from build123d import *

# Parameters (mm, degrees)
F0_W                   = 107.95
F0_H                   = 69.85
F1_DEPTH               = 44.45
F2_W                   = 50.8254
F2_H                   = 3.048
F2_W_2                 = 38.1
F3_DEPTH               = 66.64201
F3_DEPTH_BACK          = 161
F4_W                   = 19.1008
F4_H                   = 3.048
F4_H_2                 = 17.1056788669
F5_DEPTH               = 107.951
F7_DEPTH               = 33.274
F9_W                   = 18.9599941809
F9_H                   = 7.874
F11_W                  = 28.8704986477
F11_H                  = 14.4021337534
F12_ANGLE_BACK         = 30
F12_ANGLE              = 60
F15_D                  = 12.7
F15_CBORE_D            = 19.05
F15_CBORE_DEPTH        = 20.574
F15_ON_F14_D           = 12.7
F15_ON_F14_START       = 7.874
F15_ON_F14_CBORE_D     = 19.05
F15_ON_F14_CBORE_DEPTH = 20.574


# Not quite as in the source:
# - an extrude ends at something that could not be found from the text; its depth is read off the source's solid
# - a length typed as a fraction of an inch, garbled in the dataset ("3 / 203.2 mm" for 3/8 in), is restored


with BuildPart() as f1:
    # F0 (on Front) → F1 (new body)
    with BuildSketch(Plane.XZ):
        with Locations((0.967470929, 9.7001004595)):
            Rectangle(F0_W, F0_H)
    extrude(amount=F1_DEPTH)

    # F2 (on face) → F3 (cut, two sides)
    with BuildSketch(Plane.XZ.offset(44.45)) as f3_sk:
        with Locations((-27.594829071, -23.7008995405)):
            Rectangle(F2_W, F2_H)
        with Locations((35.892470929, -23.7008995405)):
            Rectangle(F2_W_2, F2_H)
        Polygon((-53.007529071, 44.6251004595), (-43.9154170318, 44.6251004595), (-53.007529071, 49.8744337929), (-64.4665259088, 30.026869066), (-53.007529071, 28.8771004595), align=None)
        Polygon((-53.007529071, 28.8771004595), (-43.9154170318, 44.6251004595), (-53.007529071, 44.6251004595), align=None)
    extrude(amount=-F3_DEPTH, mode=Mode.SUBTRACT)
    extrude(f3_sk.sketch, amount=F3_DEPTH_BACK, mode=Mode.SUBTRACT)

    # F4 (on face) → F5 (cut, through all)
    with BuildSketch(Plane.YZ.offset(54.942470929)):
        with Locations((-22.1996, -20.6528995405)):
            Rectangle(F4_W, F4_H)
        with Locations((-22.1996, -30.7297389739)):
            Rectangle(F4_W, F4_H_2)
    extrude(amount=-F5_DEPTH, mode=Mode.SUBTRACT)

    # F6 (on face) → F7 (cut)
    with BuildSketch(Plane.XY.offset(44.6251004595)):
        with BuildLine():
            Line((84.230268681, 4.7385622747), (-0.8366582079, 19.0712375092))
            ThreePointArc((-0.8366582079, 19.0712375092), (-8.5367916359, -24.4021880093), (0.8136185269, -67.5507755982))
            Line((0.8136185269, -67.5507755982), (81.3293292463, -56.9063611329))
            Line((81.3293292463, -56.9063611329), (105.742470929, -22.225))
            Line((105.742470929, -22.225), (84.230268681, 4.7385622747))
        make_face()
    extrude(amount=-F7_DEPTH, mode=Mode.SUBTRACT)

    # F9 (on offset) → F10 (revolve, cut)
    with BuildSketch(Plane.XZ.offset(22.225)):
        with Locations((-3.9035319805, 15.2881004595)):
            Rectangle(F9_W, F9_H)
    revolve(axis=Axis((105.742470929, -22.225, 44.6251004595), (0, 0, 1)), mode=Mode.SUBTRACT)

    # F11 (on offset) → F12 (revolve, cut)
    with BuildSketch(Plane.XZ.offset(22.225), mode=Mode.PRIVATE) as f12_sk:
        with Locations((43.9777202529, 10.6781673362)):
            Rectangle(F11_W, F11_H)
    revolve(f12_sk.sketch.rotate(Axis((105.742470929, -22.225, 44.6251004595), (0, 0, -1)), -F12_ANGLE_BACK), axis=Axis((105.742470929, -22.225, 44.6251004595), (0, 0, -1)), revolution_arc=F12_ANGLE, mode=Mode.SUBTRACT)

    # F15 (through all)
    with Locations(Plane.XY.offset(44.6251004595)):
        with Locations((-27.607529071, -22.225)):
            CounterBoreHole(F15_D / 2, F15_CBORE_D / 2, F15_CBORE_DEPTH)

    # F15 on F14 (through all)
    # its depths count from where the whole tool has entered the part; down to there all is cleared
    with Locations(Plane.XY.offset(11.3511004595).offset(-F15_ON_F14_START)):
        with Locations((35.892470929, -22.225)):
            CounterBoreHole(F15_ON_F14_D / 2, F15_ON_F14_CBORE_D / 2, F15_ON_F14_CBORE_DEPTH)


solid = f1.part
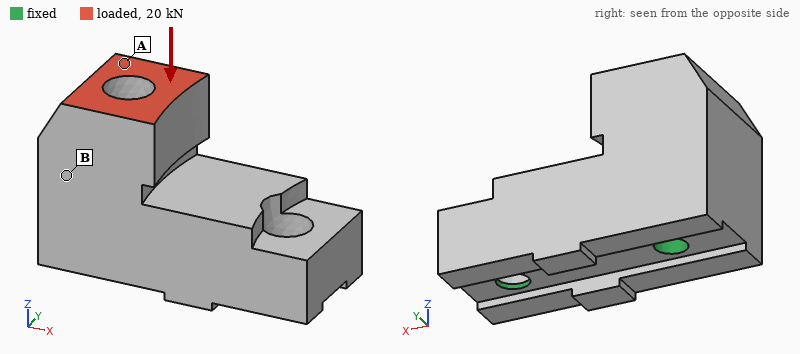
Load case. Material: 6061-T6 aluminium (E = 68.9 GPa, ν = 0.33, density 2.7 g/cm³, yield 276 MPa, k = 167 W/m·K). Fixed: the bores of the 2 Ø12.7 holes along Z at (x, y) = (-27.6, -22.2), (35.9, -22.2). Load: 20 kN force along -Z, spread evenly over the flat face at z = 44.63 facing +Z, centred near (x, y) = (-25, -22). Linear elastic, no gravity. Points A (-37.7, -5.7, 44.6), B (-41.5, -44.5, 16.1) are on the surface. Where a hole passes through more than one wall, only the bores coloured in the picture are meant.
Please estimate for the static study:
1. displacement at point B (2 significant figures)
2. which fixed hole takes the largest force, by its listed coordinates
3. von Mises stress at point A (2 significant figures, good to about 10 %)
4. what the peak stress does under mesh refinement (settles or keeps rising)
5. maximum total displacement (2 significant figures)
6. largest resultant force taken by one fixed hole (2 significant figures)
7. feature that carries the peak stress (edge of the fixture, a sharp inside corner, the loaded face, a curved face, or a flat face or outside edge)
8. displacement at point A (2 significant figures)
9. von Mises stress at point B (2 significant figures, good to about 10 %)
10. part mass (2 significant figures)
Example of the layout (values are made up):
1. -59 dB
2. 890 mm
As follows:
1. 3.6 µm
2. (-27.6, -22.2)
3. 14 MPa
4. keeps rising
5. 16 µm
6. 20 kN
7. edge of the fixture
8. 9.3 µm
9. 5.8 MPa
10. 520 g
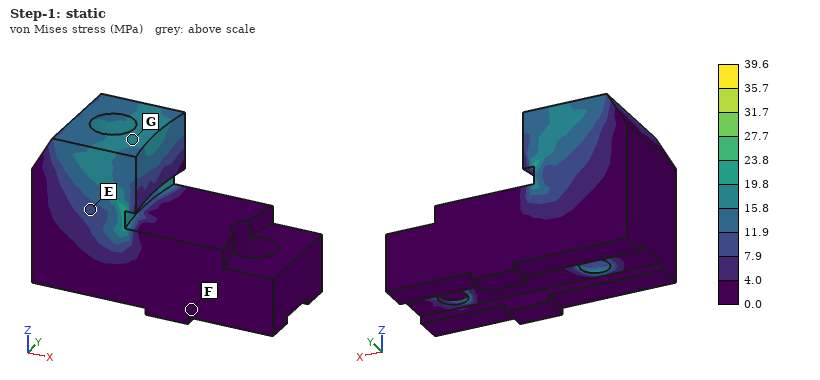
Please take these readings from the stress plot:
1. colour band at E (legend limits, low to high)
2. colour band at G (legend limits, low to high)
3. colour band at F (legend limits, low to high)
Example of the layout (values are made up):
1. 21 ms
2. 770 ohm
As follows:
1. 7.9 to 11.9 MPa
2. 15.8 to 19.8 MPa
3. 0.0 to 4.0 MPa
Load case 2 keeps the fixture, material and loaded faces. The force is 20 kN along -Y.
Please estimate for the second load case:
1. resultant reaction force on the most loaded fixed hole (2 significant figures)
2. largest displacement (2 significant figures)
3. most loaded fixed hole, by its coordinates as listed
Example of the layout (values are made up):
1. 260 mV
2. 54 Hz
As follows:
1. 20 kN
2. 68 µm
3. (-27.6, -22.2)
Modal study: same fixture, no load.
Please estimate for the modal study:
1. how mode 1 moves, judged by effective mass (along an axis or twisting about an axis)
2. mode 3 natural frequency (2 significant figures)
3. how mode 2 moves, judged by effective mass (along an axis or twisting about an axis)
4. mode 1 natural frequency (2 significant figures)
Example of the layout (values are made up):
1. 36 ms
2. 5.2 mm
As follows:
1. along Y
2. 13 kHz
3. along Z
4. 7700 Hz
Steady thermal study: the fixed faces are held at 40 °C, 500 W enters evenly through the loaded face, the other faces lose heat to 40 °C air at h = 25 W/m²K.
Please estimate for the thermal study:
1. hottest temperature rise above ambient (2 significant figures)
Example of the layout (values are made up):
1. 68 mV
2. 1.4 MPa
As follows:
1. 74 K
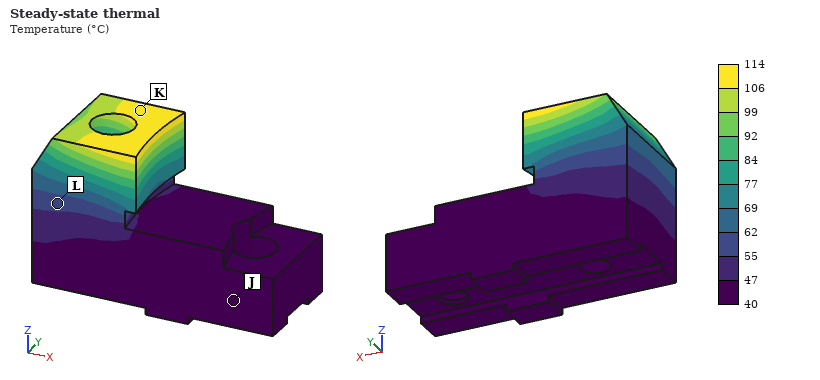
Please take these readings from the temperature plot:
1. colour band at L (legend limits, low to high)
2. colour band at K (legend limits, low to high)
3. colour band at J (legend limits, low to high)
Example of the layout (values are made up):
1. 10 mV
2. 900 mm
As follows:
1. 55 to 62 °C
2. 106 to 114 °C
3. 40 to 47 °C
